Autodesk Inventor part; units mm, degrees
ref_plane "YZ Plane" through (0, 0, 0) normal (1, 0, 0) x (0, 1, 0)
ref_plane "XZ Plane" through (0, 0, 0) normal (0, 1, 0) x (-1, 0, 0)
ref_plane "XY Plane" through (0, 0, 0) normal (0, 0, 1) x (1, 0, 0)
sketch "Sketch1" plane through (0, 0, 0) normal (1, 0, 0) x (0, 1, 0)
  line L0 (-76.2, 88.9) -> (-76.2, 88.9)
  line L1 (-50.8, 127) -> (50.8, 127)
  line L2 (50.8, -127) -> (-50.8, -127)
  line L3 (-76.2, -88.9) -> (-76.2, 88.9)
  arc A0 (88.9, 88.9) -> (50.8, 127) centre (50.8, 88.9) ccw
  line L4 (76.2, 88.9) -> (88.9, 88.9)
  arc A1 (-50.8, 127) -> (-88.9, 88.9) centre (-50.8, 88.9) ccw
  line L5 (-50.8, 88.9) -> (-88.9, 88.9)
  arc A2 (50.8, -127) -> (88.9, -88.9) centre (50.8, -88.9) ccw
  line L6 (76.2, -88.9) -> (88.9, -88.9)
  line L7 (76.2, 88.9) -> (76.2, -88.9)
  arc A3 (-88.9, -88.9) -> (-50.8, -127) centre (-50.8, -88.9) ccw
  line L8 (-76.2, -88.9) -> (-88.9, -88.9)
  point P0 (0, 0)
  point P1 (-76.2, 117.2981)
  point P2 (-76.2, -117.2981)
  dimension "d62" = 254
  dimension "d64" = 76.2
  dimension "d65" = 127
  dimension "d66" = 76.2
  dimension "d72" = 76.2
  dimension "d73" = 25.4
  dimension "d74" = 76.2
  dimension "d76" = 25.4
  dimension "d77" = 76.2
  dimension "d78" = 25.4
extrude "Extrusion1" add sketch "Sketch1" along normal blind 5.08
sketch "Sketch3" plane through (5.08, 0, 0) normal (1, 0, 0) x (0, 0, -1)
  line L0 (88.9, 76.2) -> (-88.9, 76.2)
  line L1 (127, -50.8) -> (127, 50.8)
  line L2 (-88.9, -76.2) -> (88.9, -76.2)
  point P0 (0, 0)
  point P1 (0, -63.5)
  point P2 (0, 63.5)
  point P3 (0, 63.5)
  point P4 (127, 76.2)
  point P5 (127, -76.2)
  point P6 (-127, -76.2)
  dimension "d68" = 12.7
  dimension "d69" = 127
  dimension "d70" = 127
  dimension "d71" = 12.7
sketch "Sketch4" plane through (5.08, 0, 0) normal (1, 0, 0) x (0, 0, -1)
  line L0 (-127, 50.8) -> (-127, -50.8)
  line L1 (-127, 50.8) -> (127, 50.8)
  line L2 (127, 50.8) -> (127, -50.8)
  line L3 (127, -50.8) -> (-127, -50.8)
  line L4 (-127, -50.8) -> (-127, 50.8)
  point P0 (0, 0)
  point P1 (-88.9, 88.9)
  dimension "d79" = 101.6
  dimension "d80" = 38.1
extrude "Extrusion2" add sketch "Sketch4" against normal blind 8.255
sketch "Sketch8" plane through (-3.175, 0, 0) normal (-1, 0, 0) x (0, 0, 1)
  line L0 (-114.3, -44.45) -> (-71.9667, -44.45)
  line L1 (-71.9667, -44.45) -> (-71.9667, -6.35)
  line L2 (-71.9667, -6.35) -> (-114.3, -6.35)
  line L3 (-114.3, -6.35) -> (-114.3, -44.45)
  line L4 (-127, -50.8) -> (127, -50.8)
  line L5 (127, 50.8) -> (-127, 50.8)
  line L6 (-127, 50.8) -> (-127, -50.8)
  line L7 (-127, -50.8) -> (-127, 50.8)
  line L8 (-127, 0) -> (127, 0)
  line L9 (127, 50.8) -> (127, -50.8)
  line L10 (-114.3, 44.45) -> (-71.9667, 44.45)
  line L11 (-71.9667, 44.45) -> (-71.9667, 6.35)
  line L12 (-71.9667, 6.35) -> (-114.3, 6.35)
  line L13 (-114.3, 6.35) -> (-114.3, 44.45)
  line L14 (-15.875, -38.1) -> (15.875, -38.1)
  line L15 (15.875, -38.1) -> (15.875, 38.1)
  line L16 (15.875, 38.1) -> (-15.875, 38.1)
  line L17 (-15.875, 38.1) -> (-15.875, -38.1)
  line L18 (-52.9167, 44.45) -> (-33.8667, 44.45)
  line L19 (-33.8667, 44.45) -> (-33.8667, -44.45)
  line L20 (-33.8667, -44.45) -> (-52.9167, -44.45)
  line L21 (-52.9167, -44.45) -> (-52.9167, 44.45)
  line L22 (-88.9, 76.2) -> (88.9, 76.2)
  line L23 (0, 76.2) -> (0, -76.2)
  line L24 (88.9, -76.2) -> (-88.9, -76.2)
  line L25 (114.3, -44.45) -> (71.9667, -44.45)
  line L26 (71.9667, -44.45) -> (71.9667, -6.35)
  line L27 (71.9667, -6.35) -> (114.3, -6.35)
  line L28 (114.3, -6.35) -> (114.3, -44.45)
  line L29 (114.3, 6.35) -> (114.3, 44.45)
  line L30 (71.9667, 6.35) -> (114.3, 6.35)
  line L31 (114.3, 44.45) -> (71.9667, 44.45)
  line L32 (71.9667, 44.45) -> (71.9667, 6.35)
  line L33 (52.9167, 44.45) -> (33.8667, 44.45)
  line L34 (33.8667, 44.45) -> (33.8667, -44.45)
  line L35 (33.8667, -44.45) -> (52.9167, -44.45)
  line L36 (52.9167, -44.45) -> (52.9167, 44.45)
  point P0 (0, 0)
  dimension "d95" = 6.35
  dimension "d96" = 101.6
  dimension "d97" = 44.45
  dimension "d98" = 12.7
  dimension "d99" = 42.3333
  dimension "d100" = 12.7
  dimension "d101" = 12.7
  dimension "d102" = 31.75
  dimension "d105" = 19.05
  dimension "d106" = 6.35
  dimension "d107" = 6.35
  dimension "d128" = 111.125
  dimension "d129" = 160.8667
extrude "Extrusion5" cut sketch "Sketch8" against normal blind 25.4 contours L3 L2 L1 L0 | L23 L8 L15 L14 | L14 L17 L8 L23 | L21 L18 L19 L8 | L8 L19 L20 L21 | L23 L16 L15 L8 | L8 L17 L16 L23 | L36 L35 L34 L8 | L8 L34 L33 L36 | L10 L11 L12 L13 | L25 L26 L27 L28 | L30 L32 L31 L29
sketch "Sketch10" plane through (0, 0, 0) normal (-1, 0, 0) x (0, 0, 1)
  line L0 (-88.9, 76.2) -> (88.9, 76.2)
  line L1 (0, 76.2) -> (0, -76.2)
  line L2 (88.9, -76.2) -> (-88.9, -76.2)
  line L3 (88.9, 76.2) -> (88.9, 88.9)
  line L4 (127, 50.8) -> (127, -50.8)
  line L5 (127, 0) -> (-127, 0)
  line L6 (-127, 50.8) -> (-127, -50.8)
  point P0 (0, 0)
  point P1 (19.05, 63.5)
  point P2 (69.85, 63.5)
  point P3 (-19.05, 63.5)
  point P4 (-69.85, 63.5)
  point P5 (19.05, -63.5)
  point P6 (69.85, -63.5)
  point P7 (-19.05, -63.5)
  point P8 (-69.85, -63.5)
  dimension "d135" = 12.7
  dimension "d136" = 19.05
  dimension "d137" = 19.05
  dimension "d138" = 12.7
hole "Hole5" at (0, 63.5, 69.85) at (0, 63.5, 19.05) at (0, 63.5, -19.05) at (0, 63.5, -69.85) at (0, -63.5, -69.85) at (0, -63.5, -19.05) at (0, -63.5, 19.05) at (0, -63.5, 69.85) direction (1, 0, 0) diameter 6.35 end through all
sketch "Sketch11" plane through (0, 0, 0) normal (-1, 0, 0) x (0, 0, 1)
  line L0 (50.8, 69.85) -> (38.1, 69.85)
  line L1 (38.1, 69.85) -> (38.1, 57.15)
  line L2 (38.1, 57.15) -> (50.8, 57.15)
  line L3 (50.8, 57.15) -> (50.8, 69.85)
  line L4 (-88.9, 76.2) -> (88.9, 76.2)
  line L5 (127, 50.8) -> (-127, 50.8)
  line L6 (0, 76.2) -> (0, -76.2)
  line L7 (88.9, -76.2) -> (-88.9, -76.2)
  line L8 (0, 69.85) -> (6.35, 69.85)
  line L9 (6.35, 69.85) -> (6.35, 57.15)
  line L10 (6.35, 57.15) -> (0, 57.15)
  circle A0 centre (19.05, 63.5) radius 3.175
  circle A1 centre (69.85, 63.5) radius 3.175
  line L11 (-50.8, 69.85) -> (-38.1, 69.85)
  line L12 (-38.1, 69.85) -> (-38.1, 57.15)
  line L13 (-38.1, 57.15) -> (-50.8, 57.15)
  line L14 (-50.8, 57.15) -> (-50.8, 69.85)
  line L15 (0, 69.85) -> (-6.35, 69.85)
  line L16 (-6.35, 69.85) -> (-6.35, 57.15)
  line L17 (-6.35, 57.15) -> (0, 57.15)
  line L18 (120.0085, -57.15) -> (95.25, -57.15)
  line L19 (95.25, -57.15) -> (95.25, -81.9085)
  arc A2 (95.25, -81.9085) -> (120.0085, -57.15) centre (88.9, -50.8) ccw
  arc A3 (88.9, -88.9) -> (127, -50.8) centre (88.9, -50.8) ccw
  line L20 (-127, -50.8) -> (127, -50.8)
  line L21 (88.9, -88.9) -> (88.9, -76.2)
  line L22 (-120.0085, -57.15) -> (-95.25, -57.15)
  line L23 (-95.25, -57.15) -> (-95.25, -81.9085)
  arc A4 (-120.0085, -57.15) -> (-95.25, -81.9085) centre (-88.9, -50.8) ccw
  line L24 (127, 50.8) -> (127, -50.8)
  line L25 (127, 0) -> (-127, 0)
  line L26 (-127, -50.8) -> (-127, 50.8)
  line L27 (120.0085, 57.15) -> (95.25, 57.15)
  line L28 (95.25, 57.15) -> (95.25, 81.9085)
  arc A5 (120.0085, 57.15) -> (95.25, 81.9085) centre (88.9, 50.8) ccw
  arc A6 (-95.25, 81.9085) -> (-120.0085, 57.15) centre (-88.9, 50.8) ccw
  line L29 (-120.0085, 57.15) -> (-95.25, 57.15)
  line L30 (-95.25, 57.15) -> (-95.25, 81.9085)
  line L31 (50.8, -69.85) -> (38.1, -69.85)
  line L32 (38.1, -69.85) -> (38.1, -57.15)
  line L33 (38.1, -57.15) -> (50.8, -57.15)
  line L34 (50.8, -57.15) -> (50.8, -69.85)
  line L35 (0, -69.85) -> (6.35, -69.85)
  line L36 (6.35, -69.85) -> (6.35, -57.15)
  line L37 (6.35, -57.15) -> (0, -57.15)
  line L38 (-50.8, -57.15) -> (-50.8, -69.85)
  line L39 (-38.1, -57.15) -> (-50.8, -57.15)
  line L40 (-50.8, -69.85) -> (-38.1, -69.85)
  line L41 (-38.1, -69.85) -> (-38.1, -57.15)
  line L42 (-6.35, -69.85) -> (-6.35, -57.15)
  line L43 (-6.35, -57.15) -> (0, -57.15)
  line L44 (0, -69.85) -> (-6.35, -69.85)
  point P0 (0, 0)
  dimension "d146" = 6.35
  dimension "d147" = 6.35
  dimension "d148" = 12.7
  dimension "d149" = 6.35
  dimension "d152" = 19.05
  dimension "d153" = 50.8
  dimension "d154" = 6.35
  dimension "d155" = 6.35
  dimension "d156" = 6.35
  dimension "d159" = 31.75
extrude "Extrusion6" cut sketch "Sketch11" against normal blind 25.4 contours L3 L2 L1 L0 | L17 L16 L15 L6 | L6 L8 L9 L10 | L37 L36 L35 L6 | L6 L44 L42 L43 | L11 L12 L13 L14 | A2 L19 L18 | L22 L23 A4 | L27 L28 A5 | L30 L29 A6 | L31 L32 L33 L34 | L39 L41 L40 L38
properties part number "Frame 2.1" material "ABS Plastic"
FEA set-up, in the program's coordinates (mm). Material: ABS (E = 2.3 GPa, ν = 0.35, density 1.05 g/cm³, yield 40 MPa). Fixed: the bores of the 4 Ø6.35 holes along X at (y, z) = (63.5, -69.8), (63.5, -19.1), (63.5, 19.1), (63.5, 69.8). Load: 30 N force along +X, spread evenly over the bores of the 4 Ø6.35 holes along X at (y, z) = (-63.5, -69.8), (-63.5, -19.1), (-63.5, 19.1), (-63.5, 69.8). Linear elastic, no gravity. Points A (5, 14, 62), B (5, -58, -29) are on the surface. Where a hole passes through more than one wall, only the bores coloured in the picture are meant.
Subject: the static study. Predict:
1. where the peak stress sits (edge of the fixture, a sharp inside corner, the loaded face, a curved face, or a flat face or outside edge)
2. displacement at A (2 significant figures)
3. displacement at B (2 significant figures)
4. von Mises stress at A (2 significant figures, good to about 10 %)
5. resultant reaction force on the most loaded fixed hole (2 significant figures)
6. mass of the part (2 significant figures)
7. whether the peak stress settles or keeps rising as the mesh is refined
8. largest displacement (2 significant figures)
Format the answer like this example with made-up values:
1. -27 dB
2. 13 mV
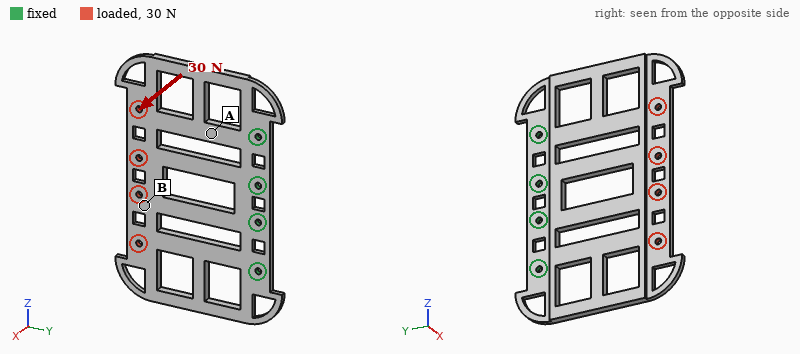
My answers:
1. edge of the fixture
2. 0.76 mm
3. 2.9 mm
4. 2.1 MPa
5. 8.5 N
6. 170 g
7. keeps rising
8. 3.7 mm
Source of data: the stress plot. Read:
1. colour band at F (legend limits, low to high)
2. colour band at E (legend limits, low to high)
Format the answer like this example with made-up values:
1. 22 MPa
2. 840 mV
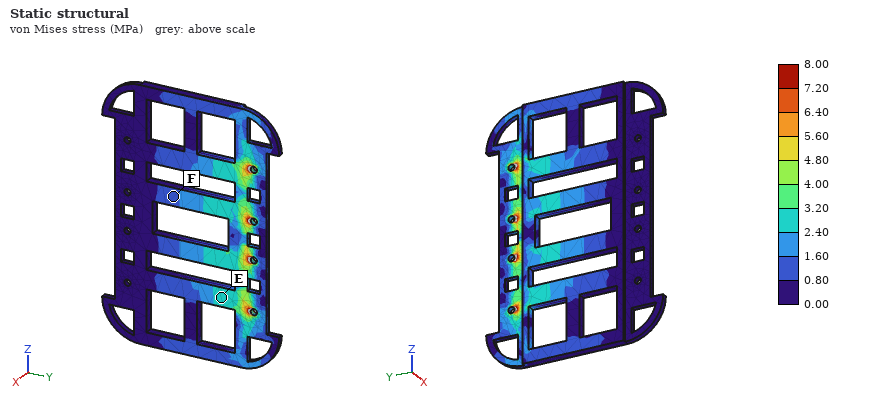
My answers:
1. 0.80 to 1.60 MPa
2. 2.40 to 3.20 MPa
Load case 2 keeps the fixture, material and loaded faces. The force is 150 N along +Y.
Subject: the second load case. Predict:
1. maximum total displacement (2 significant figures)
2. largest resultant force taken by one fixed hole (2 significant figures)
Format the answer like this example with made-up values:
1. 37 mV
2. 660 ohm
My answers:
1. 0.19 mm
2. 39 N
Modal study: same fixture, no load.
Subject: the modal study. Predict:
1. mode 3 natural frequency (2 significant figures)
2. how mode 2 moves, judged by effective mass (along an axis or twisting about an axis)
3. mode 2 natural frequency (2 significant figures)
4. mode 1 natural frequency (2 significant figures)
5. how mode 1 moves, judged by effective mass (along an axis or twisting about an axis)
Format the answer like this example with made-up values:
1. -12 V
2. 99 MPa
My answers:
1. 200 Hz
2. twisting about Y
3. 100 Hz
4. 66 Hz
5. along X
